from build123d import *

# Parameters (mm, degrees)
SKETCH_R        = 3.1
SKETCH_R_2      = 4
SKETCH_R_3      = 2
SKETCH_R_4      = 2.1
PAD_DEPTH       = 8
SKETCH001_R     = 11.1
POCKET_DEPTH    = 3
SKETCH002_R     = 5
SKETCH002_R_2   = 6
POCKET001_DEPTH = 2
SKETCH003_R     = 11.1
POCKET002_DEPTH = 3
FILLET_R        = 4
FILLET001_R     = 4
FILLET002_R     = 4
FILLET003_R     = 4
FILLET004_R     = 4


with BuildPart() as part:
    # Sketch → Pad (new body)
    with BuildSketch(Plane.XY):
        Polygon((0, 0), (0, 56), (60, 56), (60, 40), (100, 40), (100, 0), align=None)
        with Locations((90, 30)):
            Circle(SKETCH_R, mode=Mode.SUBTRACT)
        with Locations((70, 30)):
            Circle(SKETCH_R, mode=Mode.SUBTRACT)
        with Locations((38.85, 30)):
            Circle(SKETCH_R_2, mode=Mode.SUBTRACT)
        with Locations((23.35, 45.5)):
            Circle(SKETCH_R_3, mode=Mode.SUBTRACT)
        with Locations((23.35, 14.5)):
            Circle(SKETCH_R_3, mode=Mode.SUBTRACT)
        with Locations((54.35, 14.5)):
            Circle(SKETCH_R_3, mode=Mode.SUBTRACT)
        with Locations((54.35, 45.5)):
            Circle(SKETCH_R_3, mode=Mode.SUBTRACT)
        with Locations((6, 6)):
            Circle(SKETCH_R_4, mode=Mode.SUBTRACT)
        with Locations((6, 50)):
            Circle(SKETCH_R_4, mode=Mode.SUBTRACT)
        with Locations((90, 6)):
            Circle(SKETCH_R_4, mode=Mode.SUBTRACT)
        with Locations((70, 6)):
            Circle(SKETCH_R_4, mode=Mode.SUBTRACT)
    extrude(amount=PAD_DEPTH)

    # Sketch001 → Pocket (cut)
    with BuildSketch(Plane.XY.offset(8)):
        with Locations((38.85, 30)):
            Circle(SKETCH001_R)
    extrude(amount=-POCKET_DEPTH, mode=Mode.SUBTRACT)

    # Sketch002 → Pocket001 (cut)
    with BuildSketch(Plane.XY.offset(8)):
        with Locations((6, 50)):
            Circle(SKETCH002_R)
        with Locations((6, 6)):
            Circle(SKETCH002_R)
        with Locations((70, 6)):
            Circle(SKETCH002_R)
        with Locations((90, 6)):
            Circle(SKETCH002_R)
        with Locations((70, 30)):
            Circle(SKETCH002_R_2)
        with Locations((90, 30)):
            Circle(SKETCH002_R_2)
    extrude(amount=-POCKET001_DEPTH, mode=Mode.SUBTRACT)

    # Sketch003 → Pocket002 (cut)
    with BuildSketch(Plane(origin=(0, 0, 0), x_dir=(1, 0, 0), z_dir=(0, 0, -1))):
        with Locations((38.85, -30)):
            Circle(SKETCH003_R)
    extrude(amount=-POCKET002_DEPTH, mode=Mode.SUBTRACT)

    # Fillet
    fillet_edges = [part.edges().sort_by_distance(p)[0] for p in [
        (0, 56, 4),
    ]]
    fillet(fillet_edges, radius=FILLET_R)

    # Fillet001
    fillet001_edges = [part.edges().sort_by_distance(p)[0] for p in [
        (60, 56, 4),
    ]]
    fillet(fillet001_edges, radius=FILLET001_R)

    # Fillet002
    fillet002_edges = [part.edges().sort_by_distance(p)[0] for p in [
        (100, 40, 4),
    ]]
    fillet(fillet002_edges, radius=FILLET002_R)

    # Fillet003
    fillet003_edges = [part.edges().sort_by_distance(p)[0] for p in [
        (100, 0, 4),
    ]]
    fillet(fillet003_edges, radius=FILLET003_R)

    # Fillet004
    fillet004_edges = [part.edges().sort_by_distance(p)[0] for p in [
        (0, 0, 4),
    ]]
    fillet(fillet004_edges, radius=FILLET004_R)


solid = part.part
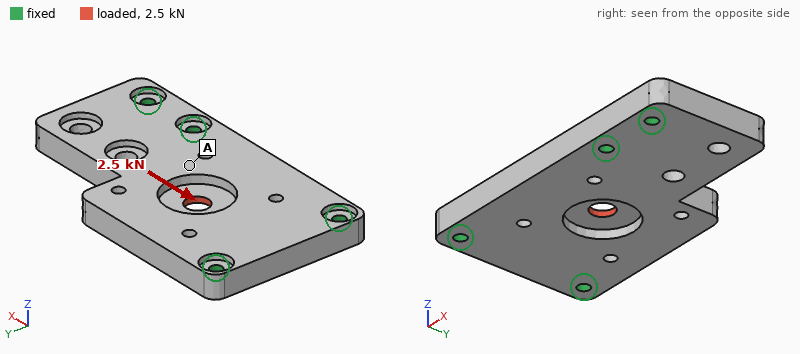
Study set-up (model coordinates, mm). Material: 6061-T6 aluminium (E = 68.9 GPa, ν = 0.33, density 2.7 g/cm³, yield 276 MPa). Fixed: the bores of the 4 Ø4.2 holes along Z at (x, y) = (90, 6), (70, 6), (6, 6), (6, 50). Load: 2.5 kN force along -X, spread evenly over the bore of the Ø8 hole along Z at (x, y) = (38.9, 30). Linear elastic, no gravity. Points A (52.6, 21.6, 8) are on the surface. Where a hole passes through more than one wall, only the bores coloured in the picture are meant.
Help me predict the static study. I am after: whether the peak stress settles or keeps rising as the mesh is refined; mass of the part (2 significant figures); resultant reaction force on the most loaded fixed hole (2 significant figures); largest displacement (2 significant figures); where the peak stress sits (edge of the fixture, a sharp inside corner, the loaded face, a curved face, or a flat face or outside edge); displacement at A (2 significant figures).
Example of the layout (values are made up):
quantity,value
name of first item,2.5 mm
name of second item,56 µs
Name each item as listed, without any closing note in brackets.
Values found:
quantity,value
whether the peak stress settles or keeps rising as the mesh is refined,keeps rising
mass of the part,94 g
resultant reaction force on the most loaded fixed hole,840 N
largest displacement,9.2 µm
where the peak stress sits,a sharp inside corner
displacement at A,3.0 µm
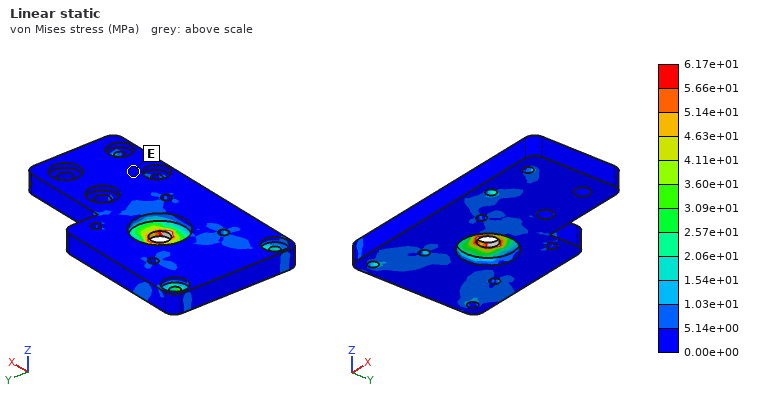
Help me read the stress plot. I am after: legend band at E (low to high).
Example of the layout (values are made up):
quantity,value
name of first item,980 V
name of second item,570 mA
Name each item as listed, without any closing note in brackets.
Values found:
quantity,value
legend band at E,0.00e+00 to 5.14e+00 MPa
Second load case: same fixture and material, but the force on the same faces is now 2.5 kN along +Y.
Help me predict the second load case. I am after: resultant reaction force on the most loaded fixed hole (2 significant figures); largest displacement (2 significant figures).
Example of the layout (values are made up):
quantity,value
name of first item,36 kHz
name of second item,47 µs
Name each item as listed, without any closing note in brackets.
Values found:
quantity,value
resultant reaction force on the most loaded fixed hole,1.1 kN
largest displacement,12 µm
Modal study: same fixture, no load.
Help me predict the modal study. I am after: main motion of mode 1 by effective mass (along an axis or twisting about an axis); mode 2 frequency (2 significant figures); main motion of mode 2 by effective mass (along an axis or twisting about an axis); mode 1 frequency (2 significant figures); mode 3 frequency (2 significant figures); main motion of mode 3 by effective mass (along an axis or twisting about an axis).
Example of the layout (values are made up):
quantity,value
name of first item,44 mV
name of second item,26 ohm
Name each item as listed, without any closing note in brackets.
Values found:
quantity,value
main motion of mode 1 by effective mass,along Z
mode 2 frequency,6500 Hz
main motion of mode 2 by effective mass,twisting about Y
mode 1 frequency,3800 Hz
mode 3 frequency,8400 Hz
main motion of mode 3 by effective mass,along Z
